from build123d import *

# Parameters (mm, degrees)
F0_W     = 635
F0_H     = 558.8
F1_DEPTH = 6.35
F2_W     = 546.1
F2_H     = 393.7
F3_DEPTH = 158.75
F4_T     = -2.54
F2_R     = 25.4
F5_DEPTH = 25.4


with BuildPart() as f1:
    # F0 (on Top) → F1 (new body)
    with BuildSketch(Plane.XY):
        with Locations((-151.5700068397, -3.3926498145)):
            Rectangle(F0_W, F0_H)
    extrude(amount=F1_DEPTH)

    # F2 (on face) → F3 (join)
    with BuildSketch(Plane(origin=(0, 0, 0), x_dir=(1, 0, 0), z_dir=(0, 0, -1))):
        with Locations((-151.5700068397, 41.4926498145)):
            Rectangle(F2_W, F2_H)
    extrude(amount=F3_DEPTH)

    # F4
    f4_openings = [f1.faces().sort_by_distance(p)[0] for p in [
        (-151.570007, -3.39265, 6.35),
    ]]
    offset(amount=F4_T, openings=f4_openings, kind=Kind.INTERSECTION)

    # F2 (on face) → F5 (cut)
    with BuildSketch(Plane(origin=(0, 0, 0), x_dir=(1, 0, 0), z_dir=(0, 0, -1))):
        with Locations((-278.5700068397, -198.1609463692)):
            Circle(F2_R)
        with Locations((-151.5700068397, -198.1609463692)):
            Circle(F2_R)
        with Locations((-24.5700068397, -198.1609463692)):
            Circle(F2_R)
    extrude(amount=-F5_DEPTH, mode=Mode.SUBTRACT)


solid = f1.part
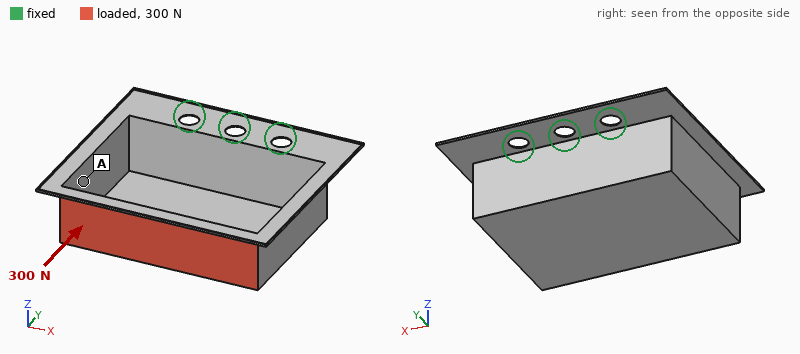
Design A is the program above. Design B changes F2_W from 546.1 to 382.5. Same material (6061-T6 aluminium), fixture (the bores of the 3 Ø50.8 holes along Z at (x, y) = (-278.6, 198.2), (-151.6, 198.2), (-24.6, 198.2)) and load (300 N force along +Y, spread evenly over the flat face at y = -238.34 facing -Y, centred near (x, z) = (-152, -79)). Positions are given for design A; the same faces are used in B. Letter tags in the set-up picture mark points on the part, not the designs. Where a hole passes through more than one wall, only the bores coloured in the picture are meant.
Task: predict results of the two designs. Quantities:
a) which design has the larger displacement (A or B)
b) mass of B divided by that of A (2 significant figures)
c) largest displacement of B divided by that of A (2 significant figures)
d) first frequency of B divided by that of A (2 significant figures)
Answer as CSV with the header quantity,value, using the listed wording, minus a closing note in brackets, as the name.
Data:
quantity,value
which design has the larger displacement,A
mass of B divided by that of A,0.92
largest displacement of B divided by that of A,0.76
first frequency of B divided by that of A,1.2
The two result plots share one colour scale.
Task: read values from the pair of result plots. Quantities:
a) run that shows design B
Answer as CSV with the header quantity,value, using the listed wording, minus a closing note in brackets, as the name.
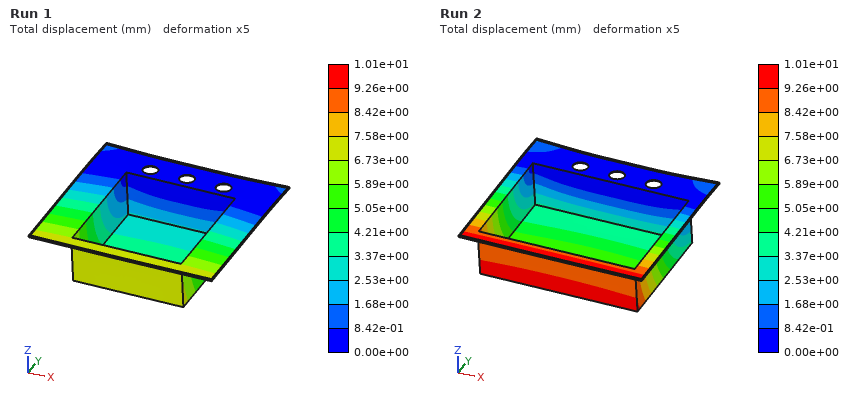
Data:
quantity,value
run that shows design B,Run 1
